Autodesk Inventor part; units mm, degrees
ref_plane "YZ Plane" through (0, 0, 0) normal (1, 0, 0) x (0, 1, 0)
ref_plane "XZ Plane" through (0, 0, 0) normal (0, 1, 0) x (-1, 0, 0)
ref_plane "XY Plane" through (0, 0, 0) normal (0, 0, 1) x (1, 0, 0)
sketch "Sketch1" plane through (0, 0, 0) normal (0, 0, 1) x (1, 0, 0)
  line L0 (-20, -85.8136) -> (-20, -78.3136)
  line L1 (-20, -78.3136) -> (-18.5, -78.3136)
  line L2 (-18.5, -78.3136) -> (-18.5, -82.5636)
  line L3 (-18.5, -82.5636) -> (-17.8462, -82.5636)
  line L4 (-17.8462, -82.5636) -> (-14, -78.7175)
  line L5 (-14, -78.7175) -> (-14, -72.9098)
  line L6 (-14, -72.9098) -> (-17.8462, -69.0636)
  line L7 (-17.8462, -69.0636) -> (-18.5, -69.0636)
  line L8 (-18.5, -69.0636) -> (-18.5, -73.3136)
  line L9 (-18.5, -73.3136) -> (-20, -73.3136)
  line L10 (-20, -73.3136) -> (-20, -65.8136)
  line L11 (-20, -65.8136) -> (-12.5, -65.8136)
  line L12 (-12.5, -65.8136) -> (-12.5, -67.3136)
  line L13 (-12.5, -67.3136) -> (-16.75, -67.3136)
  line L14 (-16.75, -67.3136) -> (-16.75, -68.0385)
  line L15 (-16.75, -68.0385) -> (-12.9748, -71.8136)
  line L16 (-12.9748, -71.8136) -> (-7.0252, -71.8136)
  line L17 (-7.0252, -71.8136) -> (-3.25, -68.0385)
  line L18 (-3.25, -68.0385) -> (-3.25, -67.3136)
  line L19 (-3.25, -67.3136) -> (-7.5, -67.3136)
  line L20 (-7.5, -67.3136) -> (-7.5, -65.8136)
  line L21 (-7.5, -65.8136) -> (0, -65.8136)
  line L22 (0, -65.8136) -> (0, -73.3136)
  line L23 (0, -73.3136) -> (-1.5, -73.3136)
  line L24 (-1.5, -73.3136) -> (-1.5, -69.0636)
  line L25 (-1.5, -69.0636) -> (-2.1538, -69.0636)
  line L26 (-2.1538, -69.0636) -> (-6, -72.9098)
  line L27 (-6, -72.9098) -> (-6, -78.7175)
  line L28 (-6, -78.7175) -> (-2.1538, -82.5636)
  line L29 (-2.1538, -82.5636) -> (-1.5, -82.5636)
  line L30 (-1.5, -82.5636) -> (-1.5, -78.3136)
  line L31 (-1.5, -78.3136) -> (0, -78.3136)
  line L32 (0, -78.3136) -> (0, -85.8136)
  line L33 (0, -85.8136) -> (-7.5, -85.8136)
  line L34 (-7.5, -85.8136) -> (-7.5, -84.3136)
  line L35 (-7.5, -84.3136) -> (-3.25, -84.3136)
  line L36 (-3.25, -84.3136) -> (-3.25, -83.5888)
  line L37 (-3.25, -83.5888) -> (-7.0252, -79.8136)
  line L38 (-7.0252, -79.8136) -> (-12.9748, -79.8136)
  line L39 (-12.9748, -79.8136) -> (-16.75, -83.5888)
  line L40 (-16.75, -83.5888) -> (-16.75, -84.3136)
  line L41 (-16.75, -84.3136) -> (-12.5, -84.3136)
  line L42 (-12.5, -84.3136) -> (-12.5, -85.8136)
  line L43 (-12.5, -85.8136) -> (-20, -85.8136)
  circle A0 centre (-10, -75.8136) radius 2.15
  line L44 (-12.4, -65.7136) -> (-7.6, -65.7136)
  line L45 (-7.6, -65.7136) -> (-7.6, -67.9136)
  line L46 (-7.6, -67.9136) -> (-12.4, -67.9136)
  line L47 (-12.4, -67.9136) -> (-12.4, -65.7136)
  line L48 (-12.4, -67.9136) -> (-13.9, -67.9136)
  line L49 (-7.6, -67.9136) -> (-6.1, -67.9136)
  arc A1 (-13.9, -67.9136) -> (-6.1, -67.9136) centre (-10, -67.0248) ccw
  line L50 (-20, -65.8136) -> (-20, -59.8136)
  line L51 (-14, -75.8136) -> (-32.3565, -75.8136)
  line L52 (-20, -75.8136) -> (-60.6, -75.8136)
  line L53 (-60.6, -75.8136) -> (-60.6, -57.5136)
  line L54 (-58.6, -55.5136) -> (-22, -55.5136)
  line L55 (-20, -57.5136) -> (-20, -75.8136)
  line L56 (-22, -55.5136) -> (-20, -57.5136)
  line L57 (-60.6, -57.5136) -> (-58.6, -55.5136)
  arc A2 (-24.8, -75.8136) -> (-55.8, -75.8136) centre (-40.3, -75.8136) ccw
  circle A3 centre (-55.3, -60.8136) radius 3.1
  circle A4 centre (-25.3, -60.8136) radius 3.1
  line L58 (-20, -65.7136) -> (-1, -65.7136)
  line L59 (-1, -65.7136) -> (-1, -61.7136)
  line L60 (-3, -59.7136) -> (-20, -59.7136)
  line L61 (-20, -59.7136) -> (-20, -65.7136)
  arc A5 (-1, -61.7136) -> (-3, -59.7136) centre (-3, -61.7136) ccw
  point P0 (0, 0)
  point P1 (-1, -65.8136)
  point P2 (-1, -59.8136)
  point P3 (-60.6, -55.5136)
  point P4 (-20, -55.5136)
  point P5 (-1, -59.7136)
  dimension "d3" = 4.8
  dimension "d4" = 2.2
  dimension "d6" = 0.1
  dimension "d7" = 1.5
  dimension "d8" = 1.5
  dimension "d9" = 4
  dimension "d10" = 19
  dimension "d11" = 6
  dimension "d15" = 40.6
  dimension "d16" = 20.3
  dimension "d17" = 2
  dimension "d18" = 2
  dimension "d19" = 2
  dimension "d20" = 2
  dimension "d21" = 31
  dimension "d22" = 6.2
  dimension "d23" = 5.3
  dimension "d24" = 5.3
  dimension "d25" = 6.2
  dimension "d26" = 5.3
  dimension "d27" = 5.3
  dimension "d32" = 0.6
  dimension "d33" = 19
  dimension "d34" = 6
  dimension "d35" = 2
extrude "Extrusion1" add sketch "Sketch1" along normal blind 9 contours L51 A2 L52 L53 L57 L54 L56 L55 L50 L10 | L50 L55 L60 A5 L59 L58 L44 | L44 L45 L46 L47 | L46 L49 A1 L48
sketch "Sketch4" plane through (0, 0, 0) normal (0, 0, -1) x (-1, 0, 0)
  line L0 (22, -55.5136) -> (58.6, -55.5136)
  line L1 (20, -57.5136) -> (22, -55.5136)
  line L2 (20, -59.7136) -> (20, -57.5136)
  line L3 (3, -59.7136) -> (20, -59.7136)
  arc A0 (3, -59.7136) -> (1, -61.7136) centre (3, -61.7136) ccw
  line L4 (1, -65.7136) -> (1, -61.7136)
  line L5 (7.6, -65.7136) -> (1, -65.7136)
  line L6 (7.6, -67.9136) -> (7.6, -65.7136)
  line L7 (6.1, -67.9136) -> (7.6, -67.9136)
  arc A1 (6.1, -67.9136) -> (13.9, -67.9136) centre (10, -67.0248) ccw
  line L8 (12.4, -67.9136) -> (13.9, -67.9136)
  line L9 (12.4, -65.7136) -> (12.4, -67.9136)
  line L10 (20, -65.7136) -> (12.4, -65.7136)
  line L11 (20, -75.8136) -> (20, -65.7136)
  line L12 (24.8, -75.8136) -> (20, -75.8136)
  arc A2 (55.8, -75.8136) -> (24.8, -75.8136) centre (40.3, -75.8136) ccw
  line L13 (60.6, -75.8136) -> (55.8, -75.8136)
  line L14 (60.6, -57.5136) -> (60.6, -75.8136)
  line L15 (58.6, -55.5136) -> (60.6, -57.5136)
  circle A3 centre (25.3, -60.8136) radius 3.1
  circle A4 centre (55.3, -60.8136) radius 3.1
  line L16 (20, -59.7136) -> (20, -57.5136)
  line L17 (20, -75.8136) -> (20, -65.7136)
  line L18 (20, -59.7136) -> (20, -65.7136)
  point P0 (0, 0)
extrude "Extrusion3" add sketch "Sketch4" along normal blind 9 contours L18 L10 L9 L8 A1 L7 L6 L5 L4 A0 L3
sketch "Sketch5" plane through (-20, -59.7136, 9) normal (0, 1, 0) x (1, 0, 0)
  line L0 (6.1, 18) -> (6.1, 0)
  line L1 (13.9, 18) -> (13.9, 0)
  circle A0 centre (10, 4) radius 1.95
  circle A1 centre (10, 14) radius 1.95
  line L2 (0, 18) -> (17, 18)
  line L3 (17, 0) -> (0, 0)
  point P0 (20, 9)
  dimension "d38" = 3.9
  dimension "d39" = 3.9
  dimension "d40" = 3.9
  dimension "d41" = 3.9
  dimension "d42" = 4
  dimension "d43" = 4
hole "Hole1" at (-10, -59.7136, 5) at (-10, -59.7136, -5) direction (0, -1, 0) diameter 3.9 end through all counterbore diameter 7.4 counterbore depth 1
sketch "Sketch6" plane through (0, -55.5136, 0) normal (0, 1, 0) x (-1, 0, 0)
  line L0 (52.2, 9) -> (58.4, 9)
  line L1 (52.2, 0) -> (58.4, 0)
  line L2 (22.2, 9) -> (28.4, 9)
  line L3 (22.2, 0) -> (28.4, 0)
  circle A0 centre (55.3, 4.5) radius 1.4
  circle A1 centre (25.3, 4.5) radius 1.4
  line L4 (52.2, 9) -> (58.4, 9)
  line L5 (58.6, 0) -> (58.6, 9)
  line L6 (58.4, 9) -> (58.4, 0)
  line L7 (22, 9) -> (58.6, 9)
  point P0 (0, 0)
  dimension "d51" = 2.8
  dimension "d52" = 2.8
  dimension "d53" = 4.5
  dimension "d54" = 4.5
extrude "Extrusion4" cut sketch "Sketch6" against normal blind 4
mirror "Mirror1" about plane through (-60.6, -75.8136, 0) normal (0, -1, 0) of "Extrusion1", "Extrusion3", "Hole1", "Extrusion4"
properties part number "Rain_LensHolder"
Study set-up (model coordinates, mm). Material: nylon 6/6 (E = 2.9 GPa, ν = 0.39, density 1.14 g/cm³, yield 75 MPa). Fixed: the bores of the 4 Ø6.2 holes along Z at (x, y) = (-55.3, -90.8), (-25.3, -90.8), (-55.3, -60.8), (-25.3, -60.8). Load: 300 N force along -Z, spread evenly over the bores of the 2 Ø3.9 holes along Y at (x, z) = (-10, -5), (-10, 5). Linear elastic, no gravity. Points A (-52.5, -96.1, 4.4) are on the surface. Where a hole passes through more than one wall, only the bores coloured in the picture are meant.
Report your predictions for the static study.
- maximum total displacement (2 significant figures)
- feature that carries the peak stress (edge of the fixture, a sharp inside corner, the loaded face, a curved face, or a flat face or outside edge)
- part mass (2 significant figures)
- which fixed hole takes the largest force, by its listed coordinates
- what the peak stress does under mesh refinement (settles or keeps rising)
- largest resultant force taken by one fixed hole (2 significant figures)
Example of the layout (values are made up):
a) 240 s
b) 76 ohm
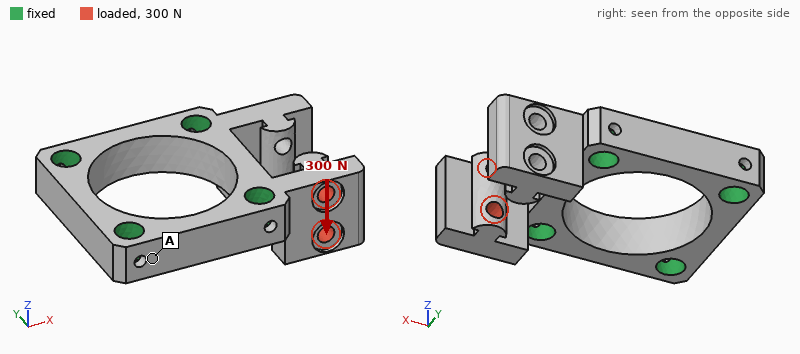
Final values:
a) 0.53 mm
b) edge of the fixture
c) 13 g
d) (-25.3, -90.8)
e) keeps rising
f) 300 N
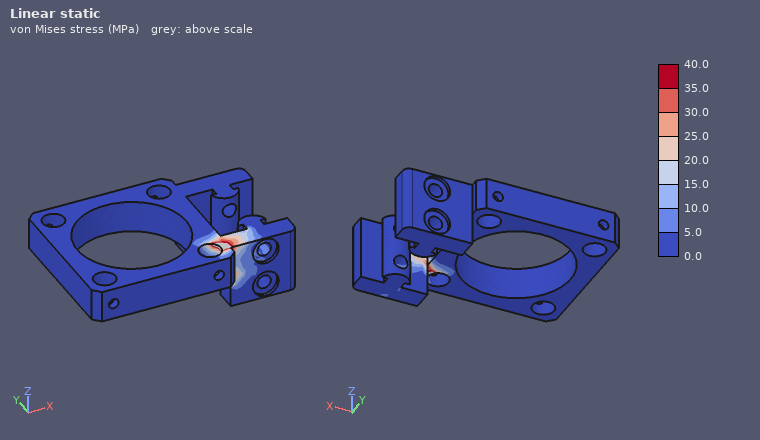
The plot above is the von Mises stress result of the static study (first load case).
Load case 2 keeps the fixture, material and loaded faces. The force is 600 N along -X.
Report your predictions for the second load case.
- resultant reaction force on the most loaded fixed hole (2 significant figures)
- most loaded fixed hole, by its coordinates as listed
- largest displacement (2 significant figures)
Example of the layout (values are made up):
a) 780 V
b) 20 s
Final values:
a) 580 N
b) (-25.3, -90.8)
c) 0.82 mm
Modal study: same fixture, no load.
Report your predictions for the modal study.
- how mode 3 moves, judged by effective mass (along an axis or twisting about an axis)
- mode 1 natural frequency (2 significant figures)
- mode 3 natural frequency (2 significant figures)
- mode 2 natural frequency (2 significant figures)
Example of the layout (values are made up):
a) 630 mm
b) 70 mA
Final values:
a) along Z
b) 2300 Hz
c) 2900 Hz
d) 2300 Hz
